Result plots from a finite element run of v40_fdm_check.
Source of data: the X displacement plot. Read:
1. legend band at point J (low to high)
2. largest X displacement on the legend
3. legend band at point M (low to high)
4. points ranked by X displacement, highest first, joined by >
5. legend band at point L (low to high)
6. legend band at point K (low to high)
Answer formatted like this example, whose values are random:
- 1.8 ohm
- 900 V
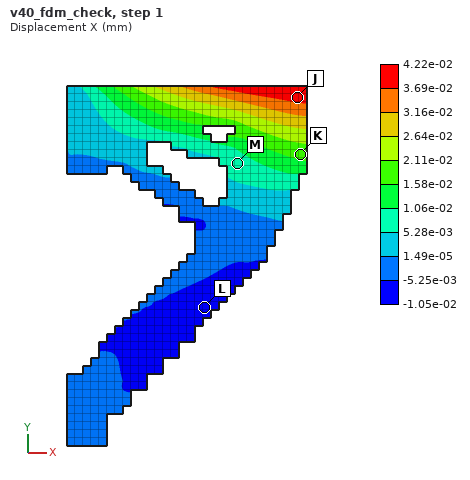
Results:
- 3.69e-02 to 4.22e-02 mm
- 4.22e-02 mm
- 5.28e-03 to 1.06e-02 mm
- J > K > M > L
- -1.05e-02 to -5.25e-03 mm
- 1.58e-02 to 2.11e-02 mm
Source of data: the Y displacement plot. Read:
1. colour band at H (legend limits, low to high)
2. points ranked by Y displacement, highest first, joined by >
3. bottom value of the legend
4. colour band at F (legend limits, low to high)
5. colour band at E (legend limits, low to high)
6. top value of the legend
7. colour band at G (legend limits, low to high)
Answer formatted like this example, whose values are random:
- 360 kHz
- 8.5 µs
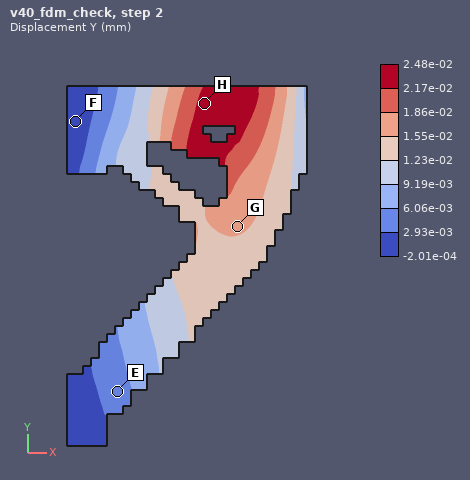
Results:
- 2.17e-02 to 2.48e-02 mm
- H > G > E > F
- -2.01e-04 mm
- -2.01e-04 to 2.93e-03 mm
- 2.93e-03 to 6.06e-03 mm
- 2.48e-02 mm
- 1.55e-02 to 1.86e-02 mm
